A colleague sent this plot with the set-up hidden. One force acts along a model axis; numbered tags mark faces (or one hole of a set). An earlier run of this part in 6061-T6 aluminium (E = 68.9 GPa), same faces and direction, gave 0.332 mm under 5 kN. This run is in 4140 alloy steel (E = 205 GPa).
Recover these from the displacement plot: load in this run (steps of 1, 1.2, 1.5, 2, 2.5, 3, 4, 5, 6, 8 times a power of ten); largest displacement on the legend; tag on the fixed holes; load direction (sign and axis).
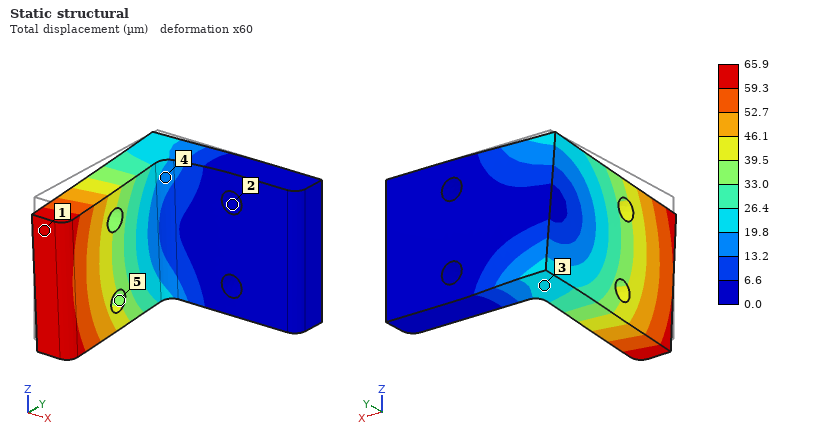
3 kN
65.9 µm
2
-Z
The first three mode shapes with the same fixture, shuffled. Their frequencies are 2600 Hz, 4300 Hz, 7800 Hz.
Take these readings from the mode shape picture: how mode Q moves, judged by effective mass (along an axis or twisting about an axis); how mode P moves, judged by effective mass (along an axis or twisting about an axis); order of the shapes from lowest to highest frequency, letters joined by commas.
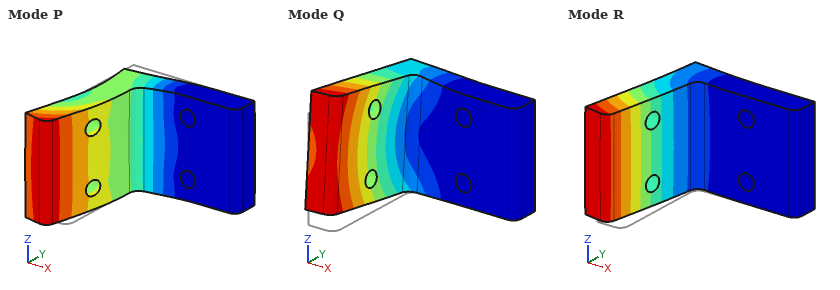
along Z
along Y
R, Q, P
